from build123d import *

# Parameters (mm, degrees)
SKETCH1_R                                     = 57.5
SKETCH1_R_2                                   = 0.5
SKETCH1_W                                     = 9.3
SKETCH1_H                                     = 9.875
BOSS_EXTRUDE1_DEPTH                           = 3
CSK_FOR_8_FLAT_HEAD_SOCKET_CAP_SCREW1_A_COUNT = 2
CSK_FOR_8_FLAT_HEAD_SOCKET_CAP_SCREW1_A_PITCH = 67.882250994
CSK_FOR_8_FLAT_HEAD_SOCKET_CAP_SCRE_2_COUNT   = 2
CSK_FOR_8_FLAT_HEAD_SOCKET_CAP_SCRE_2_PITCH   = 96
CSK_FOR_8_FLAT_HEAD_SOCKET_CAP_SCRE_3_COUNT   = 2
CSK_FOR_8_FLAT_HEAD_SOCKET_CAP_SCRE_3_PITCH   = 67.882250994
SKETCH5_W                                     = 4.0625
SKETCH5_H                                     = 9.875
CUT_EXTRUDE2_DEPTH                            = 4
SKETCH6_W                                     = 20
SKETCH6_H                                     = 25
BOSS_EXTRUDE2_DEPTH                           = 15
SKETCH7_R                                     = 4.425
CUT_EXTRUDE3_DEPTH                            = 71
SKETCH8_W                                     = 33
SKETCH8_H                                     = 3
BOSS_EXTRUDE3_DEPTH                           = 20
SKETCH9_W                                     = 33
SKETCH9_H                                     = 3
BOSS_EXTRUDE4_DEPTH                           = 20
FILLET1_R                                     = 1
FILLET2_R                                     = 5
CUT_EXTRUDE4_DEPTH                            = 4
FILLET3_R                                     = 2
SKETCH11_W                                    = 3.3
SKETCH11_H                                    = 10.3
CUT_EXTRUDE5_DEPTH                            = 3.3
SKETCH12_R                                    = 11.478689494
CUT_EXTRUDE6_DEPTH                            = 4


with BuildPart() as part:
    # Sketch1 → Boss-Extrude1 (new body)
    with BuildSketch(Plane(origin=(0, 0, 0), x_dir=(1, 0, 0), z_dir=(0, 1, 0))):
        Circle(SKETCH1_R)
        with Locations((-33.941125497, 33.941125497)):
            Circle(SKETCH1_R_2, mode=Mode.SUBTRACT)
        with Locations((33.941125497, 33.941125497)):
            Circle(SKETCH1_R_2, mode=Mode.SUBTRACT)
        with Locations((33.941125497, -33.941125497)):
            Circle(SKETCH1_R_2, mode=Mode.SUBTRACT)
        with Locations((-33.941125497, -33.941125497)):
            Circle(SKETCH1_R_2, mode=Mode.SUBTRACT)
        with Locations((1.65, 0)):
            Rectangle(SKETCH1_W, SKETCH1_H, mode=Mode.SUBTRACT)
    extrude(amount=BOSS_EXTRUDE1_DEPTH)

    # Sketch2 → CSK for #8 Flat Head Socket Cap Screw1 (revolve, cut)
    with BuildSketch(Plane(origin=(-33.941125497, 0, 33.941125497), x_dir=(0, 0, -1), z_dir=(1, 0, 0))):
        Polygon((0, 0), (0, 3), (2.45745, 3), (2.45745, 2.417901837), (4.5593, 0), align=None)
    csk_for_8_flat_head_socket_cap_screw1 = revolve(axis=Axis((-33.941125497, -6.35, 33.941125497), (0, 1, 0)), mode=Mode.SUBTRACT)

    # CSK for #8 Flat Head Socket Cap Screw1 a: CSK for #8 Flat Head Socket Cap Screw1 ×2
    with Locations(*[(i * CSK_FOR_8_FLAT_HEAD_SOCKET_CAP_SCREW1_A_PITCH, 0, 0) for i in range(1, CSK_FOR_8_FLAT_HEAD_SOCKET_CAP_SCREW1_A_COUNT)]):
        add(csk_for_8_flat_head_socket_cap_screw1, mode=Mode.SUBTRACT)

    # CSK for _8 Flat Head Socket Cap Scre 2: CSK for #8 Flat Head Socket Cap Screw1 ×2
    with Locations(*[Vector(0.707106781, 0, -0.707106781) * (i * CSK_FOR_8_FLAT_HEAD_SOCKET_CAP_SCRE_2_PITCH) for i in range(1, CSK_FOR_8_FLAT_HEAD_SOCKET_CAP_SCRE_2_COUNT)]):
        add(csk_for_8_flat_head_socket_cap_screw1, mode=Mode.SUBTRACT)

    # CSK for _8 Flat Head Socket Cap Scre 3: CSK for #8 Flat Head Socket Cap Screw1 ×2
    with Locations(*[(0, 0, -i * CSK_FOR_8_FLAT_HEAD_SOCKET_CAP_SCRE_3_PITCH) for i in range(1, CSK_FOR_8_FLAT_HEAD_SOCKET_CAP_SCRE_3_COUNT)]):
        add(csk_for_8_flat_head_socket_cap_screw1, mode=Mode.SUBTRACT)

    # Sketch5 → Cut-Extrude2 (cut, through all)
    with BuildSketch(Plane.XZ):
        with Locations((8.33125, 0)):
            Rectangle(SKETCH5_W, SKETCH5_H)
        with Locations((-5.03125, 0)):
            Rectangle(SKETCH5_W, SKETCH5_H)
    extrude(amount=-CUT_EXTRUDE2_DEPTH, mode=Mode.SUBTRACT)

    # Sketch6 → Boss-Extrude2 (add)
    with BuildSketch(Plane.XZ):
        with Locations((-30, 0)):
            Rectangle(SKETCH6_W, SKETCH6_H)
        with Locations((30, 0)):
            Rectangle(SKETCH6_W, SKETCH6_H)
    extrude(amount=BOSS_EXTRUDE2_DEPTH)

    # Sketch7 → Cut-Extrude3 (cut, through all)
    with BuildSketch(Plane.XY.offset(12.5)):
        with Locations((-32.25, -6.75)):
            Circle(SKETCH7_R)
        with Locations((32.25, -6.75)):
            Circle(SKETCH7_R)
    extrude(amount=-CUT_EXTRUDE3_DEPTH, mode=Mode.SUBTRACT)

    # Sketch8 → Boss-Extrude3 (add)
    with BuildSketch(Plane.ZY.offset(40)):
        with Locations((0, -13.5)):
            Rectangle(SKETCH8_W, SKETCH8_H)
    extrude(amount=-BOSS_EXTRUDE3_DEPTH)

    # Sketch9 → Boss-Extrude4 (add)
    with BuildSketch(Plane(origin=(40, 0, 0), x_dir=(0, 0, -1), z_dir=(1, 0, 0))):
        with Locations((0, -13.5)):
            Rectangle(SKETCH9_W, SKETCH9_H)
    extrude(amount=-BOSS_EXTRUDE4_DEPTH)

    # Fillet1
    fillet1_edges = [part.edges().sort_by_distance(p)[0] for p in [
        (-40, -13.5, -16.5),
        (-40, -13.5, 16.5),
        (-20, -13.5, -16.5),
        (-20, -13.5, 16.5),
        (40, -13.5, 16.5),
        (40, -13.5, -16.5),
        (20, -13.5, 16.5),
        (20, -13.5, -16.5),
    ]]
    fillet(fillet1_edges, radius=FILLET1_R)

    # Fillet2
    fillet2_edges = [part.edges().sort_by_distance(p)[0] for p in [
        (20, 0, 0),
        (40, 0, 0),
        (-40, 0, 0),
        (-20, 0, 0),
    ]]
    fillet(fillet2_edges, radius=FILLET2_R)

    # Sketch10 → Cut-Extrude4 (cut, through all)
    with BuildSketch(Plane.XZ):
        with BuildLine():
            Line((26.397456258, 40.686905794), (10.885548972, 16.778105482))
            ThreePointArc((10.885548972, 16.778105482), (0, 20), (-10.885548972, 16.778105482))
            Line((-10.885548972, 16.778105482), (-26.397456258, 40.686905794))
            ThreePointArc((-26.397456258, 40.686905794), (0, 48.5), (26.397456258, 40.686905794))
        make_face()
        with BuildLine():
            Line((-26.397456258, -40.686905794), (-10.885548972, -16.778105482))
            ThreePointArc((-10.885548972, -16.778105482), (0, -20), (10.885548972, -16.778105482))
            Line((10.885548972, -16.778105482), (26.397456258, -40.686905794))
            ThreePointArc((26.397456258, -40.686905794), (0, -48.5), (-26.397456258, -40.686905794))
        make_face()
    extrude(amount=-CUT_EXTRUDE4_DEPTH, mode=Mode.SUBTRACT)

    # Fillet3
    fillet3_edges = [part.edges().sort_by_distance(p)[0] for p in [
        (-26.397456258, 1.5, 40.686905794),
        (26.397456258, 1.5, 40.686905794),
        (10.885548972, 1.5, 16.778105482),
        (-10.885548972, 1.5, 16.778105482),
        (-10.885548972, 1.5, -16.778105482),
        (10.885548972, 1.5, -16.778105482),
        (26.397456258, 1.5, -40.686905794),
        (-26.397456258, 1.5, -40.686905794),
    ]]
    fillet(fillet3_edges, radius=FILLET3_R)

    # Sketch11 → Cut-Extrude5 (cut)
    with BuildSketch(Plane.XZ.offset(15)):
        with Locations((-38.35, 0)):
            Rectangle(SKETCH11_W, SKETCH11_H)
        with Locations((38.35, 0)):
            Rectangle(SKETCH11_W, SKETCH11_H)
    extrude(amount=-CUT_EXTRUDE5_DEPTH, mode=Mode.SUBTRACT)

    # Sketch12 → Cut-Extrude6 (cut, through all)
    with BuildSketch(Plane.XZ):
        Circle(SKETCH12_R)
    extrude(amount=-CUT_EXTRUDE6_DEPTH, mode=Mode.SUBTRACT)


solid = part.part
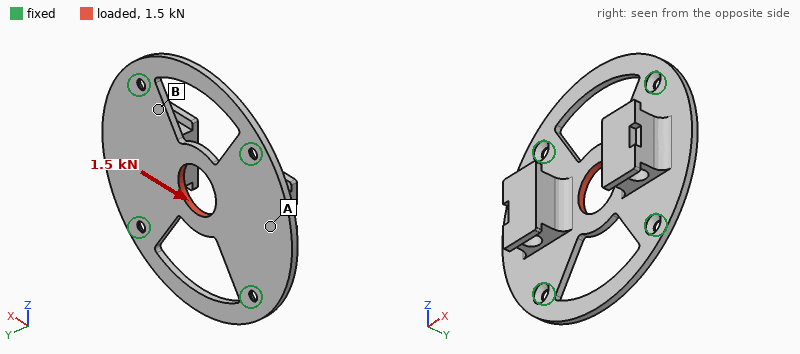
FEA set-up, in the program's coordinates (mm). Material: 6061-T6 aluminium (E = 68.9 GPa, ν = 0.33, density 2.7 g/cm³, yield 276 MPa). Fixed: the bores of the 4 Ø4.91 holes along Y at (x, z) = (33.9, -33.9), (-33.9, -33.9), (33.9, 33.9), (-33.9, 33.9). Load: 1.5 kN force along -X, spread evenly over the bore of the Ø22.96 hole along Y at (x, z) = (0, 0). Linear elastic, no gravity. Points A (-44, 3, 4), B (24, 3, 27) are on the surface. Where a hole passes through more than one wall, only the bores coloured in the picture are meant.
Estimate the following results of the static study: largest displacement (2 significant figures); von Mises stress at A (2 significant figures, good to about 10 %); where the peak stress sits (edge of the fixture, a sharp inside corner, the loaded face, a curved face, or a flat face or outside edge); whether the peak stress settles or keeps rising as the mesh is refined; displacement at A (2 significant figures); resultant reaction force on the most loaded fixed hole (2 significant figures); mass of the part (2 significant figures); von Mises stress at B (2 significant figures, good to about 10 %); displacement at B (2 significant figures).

11 µm
3.6 MPa
edge of the fixture
keeps rising
6.8 µm
380 N
97 g
9.9 MPa
5.2 µm
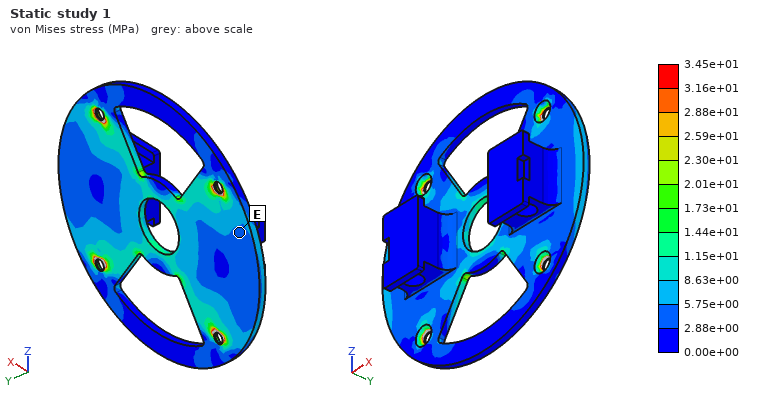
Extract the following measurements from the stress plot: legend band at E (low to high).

2.88e+00 to 5.75e+00 MPa
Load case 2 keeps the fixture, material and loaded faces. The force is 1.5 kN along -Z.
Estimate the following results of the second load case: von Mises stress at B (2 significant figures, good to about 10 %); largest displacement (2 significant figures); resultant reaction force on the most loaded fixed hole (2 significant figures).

12 MPa
13 µm
420 N
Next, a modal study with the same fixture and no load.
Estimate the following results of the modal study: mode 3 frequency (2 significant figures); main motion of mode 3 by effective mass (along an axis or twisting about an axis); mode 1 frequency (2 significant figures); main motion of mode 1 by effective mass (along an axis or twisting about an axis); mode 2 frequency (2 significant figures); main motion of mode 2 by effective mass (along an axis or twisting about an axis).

2100 Hz
twisting about X
1500 Hz
along Y
2000 Hz
along Y
